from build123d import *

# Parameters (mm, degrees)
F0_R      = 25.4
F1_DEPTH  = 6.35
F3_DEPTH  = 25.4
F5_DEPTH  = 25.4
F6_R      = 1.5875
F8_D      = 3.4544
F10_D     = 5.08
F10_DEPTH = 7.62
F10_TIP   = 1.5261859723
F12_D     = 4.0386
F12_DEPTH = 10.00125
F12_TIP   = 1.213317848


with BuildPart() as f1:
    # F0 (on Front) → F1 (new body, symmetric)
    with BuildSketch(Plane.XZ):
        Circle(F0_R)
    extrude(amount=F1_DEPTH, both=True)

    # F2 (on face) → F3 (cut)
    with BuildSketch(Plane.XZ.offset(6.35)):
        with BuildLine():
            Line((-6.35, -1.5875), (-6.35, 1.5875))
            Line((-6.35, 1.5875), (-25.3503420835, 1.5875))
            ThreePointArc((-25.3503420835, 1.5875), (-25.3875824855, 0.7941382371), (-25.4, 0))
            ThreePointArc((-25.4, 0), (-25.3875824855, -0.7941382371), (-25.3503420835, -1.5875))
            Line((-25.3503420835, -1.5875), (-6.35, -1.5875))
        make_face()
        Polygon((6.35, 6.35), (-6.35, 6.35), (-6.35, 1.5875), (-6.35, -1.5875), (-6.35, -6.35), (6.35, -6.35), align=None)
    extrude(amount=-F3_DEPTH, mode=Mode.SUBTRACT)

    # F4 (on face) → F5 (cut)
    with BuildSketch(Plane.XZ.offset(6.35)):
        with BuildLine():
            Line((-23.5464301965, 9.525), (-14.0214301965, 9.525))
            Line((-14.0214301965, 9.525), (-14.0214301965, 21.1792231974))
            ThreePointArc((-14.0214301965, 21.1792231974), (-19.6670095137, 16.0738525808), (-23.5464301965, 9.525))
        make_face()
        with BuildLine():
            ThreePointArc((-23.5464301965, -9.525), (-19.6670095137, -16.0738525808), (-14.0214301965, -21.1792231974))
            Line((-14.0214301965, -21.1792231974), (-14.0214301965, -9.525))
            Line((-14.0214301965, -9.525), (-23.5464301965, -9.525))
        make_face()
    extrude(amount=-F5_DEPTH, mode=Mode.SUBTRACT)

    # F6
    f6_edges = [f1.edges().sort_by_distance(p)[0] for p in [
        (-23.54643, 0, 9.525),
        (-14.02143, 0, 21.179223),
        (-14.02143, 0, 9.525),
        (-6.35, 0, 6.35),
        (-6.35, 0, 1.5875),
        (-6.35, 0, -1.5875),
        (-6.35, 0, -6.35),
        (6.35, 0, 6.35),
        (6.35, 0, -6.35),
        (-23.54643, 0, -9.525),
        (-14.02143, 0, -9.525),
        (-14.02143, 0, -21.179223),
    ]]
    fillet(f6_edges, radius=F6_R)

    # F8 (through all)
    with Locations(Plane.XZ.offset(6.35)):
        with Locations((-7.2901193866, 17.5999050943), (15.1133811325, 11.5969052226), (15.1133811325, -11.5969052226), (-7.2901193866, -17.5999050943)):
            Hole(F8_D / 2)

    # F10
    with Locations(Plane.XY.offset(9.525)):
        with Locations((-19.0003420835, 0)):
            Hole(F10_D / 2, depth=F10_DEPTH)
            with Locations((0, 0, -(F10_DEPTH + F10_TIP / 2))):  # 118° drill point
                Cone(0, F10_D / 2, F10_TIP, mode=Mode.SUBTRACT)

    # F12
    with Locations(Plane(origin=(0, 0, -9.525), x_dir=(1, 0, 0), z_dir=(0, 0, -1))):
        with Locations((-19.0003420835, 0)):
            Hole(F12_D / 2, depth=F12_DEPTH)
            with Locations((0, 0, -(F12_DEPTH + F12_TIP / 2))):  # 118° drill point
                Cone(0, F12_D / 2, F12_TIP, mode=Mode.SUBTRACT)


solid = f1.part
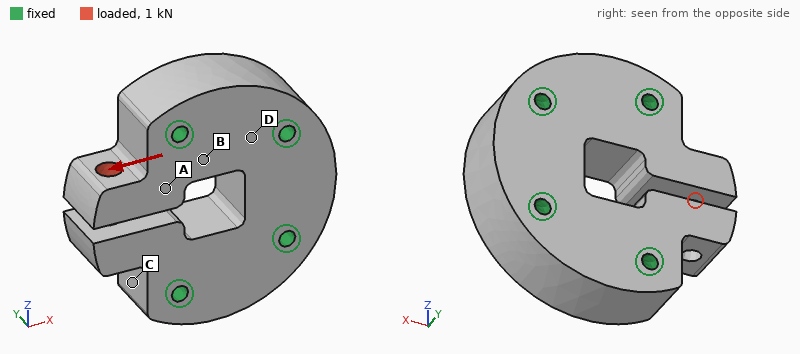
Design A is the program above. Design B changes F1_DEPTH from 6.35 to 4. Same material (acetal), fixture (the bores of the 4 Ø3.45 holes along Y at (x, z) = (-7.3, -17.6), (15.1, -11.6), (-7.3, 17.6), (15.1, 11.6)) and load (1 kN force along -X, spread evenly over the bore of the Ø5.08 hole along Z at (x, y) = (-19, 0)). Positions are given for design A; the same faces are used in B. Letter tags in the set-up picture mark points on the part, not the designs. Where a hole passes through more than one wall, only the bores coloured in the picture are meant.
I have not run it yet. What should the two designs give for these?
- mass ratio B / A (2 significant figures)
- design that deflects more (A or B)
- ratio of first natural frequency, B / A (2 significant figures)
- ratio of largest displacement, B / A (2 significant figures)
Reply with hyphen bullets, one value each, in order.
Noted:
- 0.63
- B
- 0.76
- 1.6
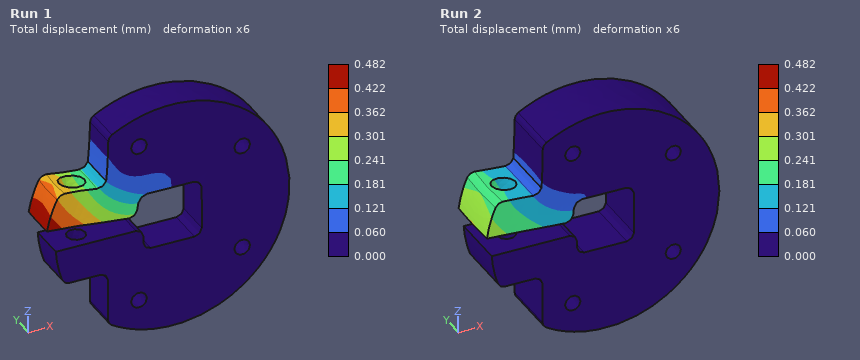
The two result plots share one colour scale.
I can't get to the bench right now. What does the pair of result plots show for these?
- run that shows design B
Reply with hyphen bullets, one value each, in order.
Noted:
- Run 1
